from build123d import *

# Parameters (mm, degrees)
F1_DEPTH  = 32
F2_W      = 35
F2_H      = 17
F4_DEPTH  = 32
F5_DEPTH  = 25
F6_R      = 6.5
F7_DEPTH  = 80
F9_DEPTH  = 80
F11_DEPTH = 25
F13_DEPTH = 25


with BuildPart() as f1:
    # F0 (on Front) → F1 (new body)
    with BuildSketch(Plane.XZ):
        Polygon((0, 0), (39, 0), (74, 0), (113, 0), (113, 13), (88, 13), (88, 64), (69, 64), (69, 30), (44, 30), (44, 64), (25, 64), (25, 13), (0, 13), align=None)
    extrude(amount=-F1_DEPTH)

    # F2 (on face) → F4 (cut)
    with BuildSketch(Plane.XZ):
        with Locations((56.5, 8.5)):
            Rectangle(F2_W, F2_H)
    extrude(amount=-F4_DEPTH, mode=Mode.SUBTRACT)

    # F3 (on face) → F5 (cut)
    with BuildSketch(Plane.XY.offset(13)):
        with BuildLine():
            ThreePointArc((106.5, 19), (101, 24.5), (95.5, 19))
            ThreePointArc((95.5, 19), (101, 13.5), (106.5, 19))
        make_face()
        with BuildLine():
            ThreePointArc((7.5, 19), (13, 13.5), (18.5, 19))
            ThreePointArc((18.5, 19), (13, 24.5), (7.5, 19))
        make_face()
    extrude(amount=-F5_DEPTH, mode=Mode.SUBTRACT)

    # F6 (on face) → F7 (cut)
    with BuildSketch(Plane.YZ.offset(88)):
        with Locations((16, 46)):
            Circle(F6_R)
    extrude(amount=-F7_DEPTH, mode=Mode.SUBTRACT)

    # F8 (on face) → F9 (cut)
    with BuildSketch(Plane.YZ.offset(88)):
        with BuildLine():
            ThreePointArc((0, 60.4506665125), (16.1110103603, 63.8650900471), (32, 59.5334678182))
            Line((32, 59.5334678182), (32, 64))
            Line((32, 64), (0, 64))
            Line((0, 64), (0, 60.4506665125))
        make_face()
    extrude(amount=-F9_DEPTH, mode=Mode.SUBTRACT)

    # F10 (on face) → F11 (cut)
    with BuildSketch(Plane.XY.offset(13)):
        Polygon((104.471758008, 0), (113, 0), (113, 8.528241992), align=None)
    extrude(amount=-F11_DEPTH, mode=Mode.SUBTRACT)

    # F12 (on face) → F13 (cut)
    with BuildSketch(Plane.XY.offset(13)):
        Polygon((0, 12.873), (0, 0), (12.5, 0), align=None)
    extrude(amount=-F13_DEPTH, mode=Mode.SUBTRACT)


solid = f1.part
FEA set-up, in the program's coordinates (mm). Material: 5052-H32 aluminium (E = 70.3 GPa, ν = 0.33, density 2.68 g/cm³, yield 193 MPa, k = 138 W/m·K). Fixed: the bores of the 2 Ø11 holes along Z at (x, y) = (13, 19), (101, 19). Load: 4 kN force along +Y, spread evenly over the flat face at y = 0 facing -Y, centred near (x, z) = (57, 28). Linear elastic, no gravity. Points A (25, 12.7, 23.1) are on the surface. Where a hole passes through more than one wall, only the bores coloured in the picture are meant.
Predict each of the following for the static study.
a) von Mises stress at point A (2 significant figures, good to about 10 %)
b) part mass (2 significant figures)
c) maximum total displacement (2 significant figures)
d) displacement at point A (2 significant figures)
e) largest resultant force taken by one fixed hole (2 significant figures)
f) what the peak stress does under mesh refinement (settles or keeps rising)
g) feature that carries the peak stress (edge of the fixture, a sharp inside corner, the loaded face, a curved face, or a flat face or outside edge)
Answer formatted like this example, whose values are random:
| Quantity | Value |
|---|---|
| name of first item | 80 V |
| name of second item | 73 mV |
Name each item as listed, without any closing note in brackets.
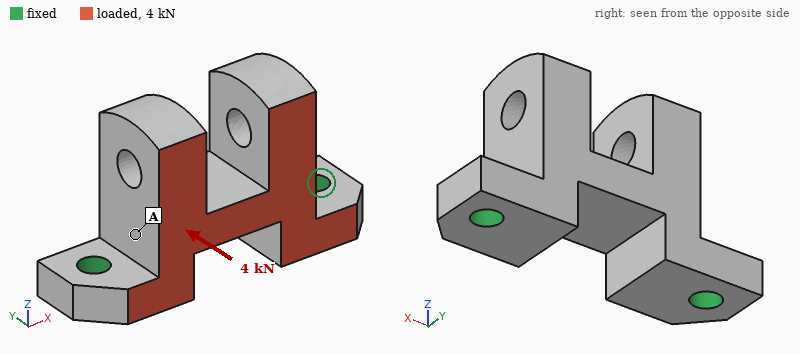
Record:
| Quantity | Value |
|---|---|
| von Mises stress at point A | 11 MPa |
| part mass | 250 g |
| maximum total displacement | 82 µm |
| displacement at point A | 26 µm |
| largest resultant force taken by one fixed hole | 2.0 kN |
| what the peak stress does under mesh refinement | keeps rising |
| feature that carries the peak stress | edge of the fixture |
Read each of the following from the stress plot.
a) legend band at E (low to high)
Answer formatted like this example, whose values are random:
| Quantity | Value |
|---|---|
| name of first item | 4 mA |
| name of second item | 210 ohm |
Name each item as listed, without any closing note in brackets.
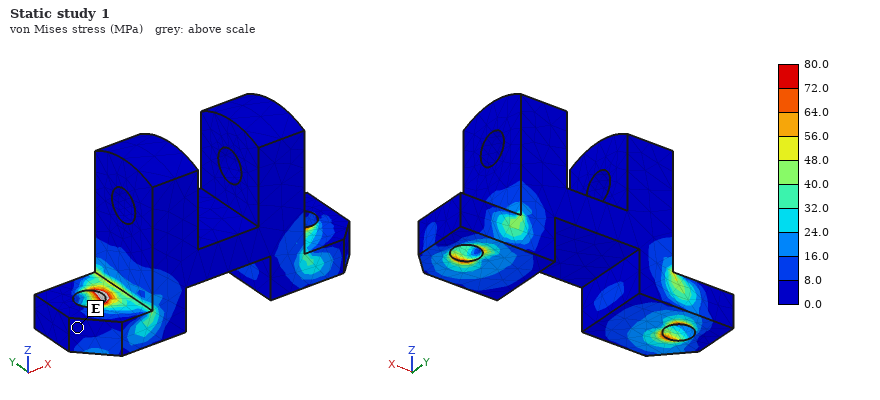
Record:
| Quantity | Value |
|---|---|
| legend band at E | 0.0 to 8.0 MPa |
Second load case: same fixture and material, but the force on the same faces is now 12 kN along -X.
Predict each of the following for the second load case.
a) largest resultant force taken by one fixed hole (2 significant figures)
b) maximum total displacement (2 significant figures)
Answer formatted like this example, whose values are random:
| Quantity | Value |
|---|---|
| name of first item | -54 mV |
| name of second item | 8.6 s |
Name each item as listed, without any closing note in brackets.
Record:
| Quantity | Value |
|---|---|
| largest resultant force taken by one fixed hole | 7.2 kN |
| maximum total displacement | 82 µm |
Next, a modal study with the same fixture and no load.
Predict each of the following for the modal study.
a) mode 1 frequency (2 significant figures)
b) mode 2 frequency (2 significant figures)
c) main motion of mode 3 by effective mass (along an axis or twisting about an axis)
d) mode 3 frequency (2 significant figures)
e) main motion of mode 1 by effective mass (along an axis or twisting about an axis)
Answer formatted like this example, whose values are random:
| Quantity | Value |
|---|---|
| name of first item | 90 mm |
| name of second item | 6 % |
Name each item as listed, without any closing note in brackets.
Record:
| Quantity | Value |
|---|---|
| mode 1 frequency | 2800 Hz |
| mode 2 frequency | 4700 Hz |
| main motion of mode 3 by effective mass | along X |
| mode 3 frequency | 5800 Hz |
| main motion of mode 1 by effective mass | along Y |
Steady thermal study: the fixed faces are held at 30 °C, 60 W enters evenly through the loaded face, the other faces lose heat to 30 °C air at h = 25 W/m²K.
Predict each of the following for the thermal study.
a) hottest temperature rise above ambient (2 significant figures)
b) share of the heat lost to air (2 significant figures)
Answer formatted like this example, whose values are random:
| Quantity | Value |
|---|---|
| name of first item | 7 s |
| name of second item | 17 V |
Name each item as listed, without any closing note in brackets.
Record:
| Quantity | Value |
|---|---|
| hottest temperature rise above ambient | 16 K |
| share of the heat lost to air | 7.1 % |
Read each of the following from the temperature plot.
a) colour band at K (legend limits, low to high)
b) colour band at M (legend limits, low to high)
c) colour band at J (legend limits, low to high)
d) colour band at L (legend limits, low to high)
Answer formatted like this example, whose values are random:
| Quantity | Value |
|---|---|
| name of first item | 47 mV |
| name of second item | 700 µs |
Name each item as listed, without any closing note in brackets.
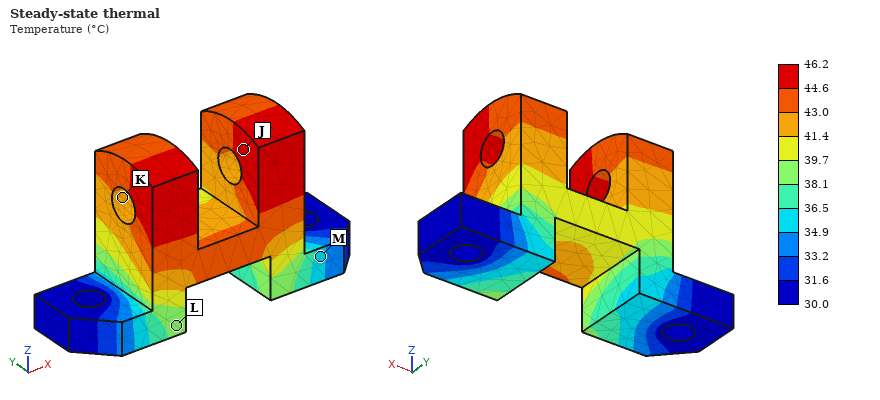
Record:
| Quantity | Value |
|---|---|
| colour band at K | 41.4 to 43.0 °C |
| colour band at M | 34.9 to 36.5 °C |
| colour band at J | 44.6 to 46.2 °C |
| colour band at L | 38.1 to 39.7 °C |
